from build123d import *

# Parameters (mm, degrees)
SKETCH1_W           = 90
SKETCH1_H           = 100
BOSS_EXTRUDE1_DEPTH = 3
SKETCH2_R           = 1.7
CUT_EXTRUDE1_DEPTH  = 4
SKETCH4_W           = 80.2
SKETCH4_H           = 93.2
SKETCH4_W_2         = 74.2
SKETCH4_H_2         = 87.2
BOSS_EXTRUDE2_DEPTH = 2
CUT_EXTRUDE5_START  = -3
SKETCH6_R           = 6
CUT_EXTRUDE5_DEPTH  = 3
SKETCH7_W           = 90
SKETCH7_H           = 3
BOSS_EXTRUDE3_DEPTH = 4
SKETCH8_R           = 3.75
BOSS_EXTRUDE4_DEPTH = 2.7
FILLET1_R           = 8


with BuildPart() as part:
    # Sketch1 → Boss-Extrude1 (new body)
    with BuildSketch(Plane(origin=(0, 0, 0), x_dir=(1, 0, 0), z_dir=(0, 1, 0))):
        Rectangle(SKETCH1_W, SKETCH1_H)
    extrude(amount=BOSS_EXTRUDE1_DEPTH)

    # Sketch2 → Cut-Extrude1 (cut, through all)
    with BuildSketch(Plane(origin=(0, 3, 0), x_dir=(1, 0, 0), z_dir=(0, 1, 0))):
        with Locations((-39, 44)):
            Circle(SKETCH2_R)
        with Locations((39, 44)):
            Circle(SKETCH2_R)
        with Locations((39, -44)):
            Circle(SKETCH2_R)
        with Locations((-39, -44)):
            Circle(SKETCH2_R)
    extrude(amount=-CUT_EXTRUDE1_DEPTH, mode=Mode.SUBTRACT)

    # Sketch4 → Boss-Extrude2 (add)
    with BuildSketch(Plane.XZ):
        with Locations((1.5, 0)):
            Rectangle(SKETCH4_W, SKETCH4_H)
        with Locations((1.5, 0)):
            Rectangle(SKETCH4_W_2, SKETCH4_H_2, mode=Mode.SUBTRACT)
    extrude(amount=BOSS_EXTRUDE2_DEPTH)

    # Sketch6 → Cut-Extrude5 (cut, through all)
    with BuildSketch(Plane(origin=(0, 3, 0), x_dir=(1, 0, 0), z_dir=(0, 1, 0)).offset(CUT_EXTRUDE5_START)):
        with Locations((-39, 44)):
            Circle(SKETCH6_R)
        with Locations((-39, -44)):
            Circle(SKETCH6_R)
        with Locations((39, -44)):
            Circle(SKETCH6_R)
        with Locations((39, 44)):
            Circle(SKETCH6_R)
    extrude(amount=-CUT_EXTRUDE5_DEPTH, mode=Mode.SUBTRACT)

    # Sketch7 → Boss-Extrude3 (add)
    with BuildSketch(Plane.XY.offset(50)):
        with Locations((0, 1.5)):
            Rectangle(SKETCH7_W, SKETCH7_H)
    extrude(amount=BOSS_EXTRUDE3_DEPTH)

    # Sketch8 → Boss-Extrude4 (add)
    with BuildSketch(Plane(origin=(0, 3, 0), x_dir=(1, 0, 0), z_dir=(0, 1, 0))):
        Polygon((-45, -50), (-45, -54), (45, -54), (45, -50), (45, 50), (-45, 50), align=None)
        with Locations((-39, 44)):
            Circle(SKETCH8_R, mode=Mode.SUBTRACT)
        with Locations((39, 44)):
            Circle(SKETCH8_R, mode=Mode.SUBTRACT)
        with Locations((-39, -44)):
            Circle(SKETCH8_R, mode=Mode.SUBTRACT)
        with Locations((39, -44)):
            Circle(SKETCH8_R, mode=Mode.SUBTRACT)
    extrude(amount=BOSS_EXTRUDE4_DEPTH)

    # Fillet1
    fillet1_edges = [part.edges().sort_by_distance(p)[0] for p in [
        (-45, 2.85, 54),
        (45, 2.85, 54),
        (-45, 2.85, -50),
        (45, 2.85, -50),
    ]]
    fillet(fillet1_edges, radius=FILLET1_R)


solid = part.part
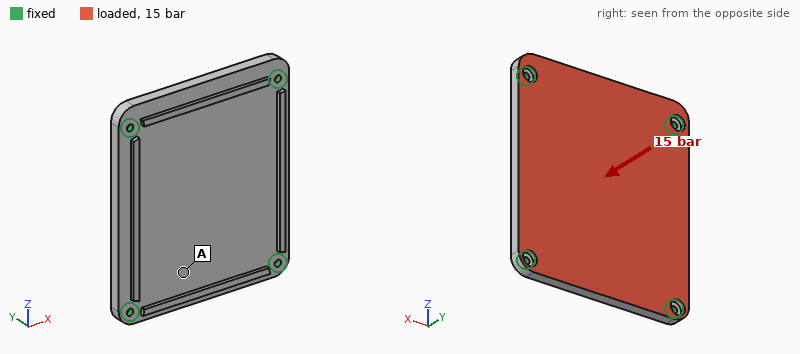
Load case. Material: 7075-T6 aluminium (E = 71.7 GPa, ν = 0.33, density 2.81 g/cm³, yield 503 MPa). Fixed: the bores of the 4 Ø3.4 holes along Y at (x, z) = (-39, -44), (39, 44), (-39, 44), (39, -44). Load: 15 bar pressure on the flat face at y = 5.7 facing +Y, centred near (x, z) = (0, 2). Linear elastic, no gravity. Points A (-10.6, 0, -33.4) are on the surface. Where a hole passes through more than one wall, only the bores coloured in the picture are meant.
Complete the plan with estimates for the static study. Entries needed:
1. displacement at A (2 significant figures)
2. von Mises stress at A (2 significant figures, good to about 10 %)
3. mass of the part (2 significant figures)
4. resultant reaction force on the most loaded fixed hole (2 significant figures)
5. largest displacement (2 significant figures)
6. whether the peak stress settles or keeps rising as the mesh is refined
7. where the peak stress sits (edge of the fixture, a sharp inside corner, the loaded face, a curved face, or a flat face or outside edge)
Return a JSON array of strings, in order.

["0.42 mm", "84 MPa", "150 g", "5.7 kN", "0.68 mm", "keeps rising", "edge of the fixture"]
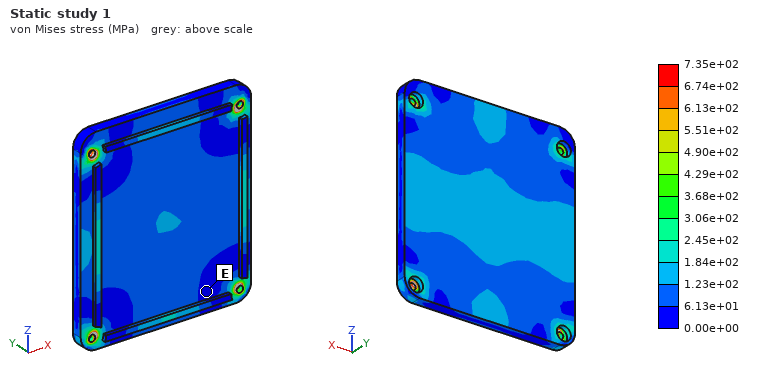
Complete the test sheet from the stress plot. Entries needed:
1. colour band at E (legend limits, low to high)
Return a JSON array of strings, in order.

["0.00e+00 to 6.13e+01 MPa"]
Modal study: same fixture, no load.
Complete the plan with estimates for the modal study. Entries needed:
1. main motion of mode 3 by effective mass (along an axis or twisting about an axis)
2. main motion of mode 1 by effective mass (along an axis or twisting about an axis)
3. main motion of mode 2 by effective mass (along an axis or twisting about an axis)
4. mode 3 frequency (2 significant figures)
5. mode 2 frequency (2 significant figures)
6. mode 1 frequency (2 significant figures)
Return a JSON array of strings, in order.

["twisting about X", "along Y", "twisting about Z", "4000 Hz", "3700 Hz", "2200 Hz"]
